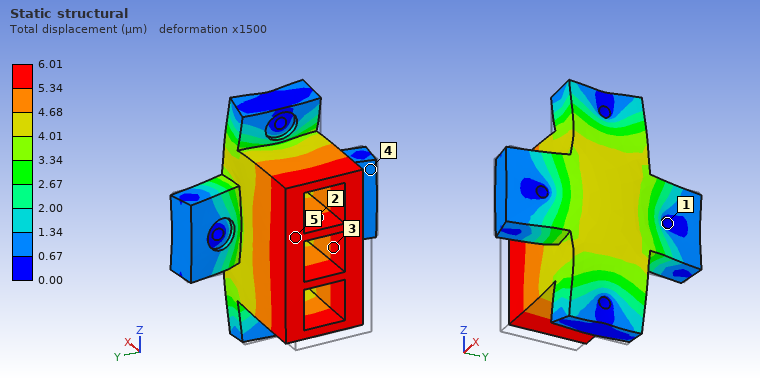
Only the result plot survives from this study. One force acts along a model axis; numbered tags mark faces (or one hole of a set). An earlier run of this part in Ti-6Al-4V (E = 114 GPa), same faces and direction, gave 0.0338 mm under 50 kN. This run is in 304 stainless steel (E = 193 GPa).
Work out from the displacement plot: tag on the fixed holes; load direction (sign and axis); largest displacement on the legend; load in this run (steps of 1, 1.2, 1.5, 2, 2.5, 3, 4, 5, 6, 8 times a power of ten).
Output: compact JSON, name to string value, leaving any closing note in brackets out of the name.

{"tag on the fixed holes": "1", "load direction": "+X", "largest displacement on the legend": "6.01 µm", "load in this run": "15 kN"}
